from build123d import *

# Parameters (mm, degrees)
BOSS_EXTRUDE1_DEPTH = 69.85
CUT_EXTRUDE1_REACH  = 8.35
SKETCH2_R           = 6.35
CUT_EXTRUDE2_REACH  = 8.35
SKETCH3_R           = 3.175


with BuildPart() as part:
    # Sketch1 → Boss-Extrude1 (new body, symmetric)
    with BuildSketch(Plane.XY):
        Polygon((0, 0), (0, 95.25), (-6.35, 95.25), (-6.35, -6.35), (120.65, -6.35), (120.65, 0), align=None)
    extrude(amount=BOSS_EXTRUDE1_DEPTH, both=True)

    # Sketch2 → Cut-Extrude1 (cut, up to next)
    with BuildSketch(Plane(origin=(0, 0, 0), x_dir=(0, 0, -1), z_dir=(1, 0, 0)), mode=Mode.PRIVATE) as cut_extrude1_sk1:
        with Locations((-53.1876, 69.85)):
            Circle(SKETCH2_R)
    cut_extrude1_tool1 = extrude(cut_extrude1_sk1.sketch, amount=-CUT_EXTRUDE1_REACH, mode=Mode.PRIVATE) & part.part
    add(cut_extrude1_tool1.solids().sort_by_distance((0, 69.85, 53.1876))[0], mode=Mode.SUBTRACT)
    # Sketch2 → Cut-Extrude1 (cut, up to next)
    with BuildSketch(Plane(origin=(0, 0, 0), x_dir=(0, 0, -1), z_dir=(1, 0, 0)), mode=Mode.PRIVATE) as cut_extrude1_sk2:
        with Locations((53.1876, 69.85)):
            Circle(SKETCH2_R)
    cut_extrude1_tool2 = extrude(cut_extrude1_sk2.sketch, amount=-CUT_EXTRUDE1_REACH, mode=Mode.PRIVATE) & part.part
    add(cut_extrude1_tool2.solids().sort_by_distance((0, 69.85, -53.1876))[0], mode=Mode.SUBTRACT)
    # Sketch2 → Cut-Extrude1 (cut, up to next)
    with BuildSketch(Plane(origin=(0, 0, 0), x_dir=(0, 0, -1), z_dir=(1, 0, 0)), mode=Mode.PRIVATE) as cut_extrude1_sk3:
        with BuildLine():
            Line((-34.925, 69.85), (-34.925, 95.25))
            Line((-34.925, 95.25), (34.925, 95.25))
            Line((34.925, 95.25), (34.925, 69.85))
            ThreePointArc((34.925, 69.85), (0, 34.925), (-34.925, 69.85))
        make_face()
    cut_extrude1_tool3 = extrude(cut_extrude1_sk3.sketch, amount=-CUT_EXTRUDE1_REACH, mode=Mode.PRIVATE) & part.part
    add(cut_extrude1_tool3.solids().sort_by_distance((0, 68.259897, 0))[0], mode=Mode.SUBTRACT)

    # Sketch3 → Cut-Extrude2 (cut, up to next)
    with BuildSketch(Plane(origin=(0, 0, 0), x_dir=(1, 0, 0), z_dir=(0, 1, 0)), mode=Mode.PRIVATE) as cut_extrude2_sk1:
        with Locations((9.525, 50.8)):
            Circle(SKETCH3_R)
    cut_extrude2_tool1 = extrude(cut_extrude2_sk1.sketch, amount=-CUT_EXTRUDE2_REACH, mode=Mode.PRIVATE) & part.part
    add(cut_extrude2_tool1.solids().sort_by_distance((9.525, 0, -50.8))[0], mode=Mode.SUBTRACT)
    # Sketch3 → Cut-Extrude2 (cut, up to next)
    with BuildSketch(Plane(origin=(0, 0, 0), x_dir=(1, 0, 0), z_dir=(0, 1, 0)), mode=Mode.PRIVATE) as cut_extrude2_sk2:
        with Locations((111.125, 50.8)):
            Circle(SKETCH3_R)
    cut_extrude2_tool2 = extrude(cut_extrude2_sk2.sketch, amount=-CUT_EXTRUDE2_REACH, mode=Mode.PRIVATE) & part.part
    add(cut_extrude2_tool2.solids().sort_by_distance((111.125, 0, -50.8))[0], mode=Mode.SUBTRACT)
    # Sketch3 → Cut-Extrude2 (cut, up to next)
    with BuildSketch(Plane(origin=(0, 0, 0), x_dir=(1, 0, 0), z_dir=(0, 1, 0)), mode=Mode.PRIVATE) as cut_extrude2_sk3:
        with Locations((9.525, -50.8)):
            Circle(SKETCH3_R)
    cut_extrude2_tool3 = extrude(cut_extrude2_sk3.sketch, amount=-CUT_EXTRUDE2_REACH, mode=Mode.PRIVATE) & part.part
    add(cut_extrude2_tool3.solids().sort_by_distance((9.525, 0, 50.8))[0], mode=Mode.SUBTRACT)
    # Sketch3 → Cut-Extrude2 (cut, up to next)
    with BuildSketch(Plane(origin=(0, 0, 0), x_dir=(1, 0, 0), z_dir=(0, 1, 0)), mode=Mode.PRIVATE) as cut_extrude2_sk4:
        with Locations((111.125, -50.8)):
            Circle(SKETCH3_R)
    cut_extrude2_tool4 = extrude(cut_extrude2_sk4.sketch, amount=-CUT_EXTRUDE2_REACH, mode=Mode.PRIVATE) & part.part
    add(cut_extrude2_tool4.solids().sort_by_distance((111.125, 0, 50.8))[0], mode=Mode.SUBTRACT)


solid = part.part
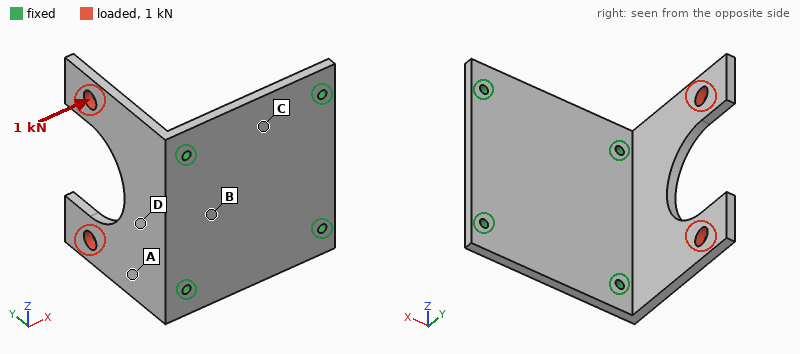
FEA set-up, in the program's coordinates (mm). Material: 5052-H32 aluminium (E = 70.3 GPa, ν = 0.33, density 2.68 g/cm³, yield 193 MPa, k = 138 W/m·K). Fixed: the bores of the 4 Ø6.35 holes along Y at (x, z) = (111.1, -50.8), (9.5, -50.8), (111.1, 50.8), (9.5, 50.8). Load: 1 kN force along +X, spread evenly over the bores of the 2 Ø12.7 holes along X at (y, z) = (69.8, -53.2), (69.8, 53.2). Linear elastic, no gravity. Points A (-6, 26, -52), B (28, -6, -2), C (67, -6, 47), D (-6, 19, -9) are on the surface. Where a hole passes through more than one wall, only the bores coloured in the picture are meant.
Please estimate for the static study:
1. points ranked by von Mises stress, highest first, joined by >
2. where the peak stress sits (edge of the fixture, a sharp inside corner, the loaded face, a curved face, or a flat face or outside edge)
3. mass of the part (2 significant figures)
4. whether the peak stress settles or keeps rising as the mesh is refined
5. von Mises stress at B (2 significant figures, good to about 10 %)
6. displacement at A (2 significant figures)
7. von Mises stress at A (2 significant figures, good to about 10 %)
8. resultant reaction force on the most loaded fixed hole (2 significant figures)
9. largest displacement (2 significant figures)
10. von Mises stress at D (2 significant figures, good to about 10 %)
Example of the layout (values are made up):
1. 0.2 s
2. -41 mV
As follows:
1. A > D > B > C
2. edge of the fixture
3. 460 g
4. keeps rising
5. 20 MPa
6. 0.31 mm
7. 54 MPa
8. 450 N
9. 1.6 mm
10. 36 MPa
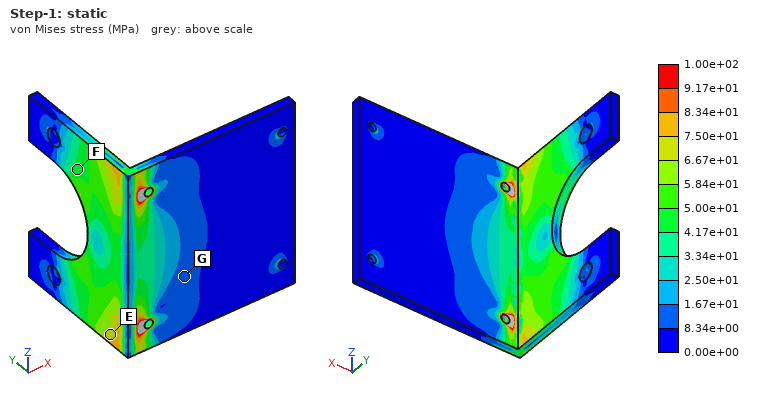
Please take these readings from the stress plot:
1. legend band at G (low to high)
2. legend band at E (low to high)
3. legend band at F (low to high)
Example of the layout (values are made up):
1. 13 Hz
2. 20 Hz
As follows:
1. 8.34e+00 to 1.67e+01 MPa
2. 6.67e+01 to 7.50e+01 MPa
3. 4.17e+01 to 5.00e+01 MPa
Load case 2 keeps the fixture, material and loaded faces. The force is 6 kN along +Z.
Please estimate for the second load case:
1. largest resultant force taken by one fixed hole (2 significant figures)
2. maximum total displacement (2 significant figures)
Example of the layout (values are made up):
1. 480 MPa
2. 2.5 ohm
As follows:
1. 5.1 kN
2. 0.40 mm
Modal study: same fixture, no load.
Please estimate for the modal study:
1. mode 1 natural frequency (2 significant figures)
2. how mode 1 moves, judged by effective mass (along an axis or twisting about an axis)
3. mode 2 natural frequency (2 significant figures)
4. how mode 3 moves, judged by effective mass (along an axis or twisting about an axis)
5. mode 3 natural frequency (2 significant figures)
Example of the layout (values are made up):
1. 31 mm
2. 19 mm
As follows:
1. 580 Hz
2. along X
3. 690 Hz
4. along Y
5. 2200 Hz
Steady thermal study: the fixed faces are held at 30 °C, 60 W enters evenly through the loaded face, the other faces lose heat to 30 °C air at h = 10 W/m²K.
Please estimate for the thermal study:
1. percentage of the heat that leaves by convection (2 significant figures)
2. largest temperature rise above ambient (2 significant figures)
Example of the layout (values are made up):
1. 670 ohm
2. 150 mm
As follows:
1. 15 %
2. 65 K
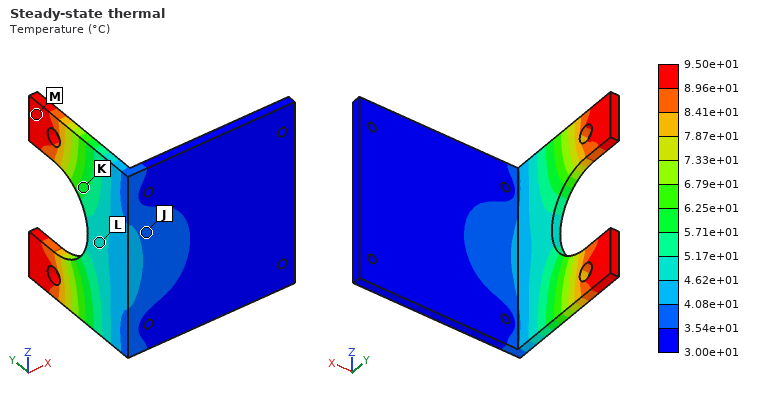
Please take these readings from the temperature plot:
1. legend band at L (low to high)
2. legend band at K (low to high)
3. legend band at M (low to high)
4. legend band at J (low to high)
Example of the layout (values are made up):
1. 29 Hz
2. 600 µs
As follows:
1. 4.62e+01 to 5.17e+01 °C
2. 5.71e+01 to 6.25e+01 °C
3. 8.96e+01 to 9.50e+01 °C
4. 3.54e+01 to 4.08e+01 °C
